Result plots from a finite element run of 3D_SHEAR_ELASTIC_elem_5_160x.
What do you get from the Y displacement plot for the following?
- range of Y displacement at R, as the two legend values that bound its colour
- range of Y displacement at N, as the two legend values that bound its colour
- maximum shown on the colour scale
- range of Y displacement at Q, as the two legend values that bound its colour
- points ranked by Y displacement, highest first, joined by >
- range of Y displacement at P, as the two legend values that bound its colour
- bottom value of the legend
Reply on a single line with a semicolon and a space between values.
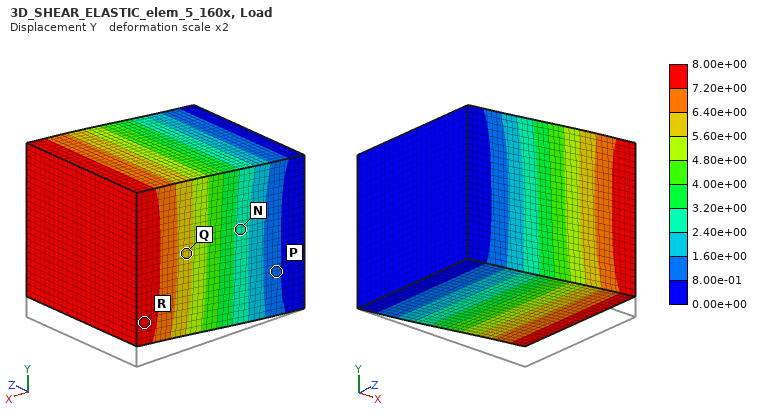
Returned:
7.20e+00 to 8.00e+00; 2.40e+00 to 3.20e+00; 8.00e+00; 5.60e+00 to 6.40e+00; R > Q > N > P; 8.00e-01 to 1.60e+00; 0.00e+00
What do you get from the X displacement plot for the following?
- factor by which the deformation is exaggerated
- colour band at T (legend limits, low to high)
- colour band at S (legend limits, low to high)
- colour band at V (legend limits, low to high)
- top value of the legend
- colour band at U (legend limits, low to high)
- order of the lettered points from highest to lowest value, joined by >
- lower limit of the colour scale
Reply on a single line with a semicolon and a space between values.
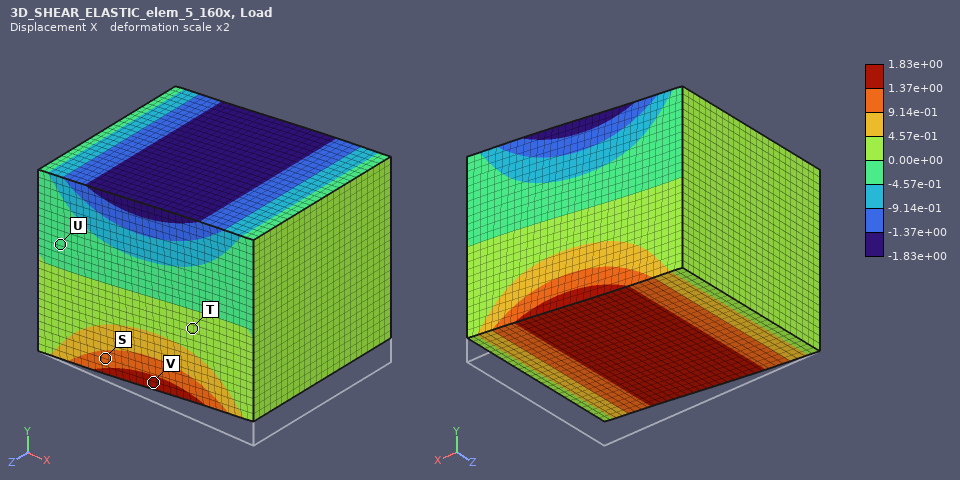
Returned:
2; 0.00e+00 to 4.57e-01; 9.14e-01 to 1.37e+00; 1.37e+00 to 1.83e+00; 1.83e+00; -4.57e-01 to 0.00e+00; V > S > T > U; -1.83e+00
